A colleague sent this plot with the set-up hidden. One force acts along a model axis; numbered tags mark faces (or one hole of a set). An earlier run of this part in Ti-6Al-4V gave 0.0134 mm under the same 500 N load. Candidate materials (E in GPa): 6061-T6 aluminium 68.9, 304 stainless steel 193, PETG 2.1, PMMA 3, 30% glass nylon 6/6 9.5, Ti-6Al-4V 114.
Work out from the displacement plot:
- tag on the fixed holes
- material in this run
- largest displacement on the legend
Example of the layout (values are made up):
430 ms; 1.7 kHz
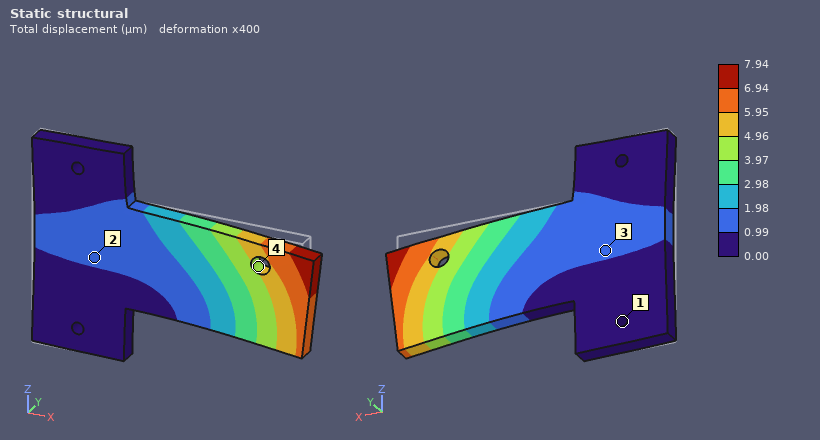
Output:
1; 304 stainless steel; 7.94 µm
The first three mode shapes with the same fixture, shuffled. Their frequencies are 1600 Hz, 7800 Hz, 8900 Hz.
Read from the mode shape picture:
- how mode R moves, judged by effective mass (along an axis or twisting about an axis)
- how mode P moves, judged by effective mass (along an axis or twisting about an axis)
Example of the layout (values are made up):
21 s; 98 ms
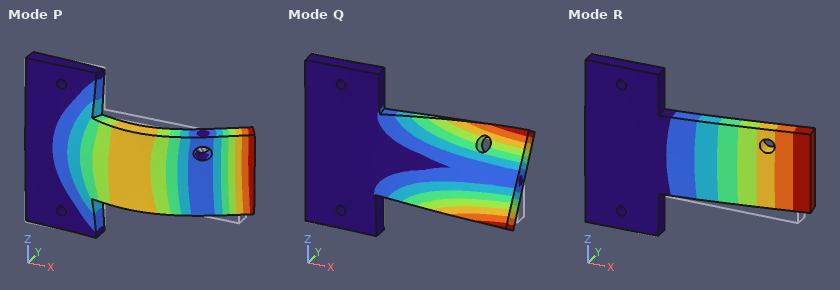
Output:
along Y; along Y
